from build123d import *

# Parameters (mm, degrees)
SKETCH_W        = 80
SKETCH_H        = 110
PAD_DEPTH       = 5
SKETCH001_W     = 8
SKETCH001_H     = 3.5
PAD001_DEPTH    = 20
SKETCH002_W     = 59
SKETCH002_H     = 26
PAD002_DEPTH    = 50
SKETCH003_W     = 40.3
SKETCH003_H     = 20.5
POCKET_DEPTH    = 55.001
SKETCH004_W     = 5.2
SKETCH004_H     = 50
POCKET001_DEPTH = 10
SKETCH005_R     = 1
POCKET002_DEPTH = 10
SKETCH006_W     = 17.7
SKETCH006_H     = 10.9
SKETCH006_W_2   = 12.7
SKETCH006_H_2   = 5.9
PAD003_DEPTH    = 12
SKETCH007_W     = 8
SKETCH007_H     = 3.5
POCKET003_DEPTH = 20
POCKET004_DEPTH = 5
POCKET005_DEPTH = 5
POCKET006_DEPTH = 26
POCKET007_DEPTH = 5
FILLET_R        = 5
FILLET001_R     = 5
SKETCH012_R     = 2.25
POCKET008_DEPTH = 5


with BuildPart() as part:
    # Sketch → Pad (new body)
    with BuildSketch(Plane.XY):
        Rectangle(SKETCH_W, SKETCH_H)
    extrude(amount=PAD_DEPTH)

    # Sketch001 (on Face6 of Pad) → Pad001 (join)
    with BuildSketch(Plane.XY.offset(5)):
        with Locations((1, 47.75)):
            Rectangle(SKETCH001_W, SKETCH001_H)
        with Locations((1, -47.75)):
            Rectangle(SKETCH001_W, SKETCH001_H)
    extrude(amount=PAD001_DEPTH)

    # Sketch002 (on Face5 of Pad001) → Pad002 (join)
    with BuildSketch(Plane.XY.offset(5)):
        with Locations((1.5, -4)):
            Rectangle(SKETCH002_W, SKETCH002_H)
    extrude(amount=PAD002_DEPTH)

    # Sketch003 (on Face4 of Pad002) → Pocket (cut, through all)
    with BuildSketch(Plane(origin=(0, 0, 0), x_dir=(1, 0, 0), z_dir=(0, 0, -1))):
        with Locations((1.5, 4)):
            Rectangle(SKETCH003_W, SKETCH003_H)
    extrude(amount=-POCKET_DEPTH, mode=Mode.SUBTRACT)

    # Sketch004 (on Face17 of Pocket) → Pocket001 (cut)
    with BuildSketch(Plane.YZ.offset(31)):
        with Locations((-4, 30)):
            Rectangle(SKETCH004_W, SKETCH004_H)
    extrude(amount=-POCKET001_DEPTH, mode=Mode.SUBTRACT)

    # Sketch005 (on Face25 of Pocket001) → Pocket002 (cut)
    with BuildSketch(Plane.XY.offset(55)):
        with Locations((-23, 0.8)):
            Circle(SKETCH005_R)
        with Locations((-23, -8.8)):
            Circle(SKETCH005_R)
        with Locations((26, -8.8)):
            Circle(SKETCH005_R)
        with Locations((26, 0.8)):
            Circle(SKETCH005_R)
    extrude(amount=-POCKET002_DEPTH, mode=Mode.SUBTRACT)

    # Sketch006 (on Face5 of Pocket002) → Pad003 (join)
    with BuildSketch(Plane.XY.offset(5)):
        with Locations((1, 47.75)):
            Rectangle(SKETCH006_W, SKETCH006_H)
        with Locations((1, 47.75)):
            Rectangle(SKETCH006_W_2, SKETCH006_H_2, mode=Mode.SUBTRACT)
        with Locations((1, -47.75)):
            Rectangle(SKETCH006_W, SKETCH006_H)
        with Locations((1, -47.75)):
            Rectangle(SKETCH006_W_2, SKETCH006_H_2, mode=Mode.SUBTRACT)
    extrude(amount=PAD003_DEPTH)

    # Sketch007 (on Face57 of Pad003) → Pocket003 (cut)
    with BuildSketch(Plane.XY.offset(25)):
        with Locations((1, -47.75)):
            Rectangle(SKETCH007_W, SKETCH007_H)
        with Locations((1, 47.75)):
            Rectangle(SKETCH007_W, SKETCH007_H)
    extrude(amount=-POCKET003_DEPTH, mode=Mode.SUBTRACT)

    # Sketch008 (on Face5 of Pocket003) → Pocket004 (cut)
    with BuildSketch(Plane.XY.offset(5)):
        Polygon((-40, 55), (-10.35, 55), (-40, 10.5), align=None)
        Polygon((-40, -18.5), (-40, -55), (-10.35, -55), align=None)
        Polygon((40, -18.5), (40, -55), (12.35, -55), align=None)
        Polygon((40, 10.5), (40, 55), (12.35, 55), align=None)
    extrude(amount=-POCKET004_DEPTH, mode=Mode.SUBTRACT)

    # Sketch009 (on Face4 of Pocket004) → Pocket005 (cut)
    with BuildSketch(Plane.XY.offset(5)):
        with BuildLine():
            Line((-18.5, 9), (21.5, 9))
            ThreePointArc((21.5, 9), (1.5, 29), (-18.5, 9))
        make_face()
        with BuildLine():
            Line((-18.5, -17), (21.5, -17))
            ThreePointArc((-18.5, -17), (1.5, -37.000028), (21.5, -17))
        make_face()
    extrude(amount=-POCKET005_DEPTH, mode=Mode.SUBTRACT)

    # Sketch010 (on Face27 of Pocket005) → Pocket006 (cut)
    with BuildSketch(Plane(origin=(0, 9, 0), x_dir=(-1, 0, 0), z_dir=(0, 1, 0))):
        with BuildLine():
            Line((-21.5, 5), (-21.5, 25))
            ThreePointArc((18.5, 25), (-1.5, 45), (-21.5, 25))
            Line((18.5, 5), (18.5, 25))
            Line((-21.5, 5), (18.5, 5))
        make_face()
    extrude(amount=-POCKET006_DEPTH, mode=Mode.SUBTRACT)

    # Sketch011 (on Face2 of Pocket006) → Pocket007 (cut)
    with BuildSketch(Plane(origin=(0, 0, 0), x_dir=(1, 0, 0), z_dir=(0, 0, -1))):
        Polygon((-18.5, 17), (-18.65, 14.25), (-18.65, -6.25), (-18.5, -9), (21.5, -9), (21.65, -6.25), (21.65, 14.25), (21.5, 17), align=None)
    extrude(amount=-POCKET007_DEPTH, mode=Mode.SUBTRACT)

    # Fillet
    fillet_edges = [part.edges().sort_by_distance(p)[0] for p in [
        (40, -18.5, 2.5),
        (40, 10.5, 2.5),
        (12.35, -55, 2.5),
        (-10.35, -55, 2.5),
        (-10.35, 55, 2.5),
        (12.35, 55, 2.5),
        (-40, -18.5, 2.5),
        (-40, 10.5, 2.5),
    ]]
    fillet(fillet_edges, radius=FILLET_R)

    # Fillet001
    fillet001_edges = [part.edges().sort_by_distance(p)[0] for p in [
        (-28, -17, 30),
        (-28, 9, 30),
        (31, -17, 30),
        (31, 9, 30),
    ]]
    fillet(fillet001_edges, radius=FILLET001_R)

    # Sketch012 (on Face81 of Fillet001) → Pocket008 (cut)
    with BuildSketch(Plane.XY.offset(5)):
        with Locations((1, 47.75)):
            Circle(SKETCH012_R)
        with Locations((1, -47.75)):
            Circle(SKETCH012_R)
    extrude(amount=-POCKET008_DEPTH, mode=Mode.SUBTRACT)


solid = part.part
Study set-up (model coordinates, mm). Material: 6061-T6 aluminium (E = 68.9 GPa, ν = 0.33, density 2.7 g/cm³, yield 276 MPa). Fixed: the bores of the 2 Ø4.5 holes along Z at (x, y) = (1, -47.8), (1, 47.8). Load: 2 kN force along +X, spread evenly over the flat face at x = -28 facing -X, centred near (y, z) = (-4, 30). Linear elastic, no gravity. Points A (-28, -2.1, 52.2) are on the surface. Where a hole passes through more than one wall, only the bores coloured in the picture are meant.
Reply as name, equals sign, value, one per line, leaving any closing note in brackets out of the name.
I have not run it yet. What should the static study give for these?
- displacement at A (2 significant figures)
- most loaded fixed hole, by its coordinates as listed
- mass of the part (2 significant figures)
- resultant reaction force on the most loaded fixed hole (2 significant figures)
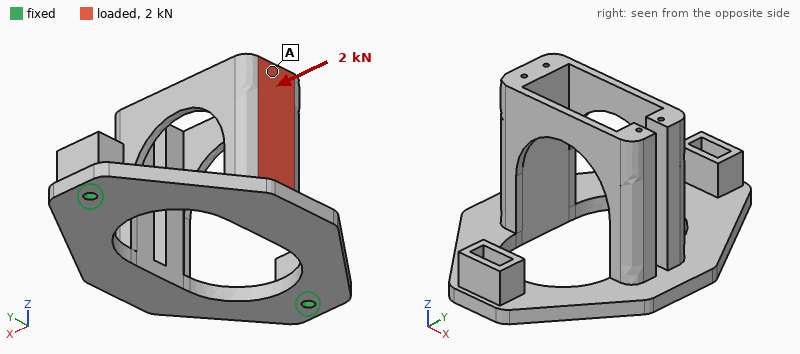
displacement at A = 1.3 mm
most loaded fixed hole, by its coordinates as listed = (1, -47.8)
mass of the part = 130 g
resultant reaction force on the most loaded fixed hole = 1.1 kN
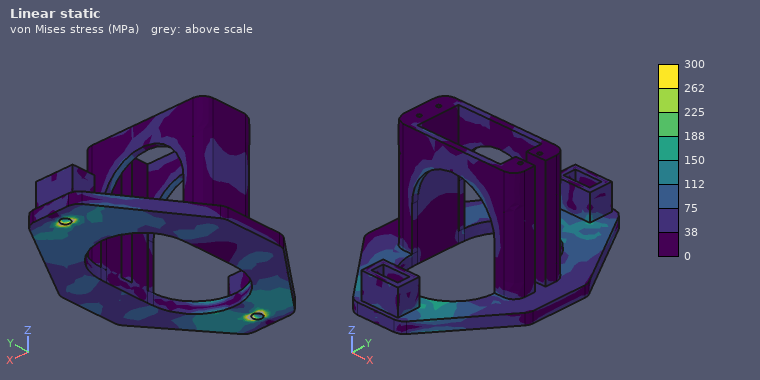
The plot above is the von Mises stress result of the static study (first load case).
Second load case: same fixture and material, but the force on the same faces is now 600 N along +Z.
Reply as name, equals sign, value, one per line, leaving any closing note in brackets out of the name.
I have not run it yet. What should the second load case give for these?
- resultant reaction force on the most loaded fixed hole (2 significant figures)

resultant reaction force on the most loaded fixed hole = 340 N
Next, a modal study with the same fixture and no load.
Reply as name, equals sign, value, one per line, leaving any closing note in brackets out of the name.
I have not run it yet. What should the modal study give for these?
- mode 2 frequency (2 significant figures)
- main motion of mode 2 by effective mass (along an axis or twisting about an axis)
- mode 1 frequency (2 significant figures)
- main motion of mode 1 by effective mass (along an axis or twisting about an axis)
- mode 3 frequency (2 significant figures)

mode 2 frequency = 1200 Hz
main motion of mode 2 by effective mass = along Z
mode 1 frequency = 710 Hz
main motion of mode 1 by effective mass = along X
mode 3 frequency = 1400 Hz
